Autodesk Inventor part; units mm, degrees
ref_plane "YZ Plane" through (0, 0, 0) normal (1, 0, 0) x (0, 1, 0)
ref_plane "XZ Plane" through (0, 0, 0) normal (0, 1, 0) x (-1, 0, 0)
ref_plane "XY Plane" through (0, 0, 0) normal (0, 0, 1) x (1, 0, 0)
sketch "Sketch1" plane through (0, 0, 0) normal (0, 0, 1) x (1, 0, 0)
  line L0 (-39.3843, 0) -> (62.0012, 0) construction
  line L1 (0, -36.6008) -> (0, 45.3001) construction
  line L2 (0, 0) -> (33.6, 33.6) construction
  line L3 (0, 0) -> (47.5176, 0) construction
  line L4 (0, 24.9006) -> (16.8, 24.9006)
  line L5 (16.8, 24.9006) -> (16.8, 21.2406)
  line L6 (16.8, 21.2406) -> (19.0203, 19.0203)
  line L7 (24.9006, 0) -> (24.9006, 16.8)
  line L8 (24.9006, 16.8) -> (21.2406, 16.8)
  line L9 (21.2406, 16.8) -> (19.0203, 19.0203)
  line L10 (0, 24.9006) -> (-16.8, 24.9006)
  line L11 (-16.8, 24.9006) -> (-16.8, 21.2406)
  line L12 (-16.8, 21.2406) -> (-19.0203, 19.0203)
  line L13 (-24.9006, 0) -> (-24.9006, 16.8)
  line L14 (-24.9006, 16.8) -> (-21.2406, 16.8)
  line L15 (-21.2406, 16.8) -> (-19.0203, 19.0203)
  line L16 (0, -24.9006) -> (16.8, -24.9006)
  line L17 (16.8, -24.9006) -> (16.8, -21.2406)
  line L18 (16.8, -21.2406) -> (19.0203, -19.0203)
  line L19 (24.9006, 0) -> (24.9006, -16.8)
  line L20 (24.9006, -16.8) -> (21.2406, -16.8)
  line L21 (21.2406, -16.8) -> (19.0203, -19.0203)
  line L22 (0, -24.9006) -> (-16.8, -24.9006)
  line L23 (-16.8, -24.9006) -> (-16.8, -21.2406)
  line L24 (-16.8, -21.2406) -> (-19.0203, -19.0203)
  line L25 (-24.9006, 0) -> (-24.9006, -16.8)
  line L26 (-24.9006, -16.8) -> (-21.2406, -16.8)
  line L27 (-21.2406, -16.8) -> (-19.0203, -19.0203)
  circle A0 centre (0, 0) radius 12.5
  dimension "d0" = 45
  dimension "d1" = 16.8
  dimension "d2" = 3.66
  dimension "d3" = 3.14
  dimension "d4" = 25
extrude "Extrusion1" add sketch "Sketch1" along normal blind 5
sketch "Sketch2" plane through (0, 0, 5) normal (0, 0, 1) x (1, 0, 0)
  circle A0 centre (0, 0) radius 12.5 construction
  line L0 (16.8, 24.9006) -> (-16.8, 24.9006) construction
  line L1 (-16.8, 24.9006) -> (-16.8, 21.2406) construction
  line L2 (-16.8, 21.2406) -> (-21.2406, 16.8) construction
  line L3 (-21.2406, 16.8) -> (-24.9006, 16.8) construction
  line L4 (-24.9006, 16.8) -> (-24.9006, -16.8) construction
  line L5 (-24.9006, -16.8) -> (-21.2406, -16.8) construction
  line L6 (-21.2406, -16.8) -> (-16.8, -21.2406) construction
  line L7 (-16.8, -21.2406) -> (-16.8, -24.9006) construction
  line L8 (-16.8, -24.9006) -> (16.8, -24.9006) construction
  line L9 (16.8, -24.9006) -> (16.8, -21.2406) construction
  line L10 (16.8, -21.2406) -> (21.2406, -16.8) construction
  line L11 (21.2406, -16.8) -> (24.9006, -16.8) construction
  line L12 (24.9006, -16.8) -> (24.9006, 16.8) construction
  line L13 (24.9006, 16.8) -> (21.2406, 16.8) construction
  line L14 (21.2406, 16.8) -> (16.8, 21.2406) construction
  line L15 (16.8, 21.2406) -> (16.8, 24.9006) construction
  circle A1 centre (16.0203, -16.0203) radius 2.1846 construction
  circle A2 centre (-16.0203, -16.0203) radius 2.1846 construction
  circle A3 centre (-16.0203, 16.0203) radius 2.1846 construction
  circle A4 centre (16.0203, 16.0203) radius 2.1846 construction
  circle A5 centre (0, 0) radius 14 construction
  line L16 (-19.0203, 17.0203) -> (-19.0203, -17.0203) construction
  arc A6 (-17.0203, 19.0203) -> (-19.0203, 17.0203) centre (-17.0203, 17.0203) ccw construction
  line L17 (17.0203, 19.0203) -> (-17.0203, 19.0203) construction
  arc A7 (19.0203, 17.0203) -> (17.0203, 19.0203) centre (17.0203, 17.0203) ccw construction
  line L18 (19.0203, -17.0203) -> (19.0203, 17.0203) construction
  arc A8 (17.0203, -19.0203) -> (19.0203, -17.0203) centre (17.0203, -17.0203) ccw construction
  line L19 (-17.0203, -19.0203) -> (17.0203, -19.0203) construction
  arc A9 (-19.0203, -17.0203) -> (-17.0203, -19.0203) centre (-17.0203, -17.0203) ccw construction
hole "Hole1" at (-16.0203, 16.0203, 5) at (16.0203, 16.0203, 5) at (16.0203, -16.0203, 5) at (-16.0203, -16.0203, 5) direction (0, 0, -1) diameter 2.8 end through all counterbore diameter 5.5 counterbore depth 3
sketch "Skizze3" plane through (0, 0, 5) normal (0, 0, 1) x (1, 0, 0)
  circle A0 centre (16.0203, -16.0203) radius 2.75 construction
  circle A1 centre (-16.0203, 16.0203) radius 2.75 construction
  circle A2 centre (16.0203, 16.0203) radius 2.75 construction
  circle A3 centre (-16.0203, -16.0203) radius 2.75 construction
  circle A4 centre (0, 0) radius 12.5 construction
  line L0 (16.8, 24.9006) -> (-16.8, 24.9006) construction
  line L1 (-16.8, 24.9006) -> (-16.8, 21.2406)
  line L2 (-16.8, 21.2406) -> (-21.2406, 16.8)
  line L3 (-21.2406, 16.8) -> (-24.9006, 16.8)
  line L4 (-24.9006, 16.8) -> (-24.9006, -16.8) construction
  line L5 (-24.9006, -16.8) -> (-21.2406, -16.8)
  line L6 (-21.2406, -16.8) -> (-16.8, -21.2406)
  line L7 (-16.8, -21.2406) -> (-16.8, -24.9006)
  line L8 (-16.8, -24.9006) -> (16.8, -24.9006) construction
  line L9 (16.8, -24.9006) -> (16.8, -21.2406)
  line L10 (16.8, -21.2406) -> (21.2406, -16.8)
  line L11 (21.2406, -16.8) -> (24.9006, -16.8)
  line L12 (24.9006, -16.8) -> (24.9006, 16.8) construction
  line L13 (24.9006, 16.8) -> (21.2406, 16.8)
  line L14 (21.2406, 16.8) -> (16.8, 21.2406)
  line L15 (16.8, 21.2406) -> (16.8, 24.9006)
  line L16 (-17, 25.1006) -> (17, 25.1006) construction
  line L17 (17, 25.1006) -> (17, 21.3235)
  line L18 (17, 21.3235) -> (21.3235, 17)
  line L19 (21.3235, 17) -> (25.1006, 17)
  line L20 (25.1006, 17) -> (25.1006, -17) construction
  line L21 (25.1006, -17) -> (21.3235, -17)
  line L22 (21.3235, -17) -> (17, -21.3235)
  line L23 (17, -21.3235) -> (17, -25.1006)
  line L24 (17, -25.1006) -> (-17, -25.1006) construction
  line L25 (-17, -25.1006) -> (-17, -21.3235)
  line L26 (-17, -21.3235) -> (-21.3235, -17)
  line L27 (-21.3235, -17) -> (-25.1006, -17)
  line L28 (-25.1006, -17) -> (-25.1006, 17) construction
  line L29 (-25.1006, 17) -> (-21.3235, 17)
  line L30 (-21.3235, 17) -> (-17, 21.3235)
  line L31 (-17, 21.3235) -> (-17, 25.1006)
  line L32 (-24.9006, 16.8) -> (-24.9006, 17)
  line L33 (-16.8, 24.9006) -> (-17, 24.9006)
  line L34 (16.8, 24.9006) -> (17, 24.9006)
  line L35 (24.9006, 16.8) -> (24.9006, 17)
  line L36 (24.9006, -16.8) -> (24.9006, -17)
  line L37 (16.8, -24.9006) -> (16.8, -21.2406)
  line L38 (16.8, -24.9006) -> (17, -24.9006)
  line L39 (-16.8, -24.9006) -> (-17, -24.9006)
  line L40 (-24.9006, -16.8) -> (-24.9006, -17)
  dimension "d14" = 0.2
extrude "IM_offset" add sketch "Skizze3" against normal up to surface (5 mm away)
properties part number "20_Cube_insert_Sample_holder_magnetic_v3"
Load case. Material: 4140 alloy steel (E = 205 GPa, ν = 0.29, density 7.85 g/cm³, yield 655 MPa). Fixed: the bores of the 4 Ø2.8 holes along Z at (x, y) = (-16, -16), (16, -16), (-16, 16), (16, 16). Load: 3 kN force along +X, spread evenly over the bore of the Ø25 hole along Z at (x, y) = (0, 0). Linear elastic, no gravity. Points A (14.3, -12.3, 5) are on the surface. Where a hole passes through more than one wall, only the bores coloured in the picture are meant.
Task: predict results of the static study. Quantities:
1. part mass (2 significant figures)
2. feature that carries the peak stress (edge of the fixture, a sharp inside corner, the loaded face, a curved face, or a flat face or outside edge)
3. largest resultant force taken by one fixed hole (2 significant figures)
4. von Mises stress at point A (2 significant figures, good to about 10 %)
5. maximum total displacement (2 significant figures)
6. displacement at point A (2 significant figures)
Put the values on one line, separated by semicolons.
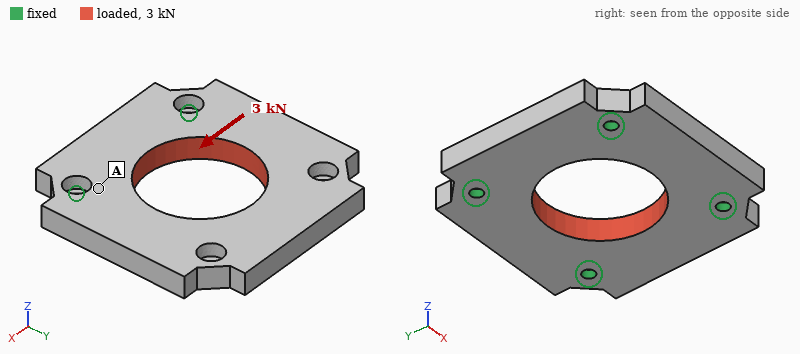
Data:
67 g; edge of the fixture; 750 N; 12 MPa; 2.7 µm; 1.4 µm
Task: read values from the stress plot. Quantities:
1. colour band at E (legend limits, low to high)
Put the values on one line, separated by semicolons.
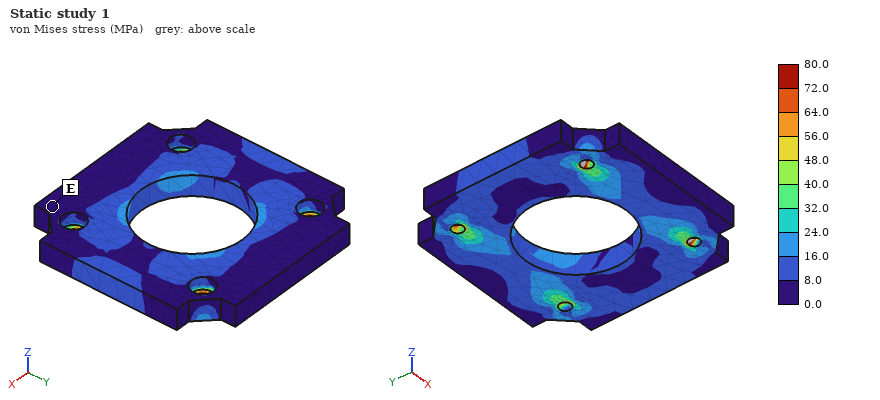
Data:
0.0 to 8.0 MPa
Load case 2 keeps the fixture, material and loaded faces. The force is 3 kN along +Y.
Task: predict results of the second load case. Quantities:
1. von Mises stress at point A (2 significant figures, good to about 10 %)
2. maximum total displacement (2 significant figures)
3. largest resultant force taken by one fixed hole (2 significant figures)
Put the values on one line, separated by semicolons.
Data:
8.6 MPa; 2.7 µm; 750 N
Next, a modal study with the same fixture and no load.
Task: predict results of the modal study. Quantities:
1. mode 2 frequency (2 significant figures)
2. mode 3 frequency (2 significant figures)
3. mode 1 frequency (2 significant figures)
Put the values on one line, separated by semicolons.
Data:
15 kHz; 15 kHz; 12 kHz
